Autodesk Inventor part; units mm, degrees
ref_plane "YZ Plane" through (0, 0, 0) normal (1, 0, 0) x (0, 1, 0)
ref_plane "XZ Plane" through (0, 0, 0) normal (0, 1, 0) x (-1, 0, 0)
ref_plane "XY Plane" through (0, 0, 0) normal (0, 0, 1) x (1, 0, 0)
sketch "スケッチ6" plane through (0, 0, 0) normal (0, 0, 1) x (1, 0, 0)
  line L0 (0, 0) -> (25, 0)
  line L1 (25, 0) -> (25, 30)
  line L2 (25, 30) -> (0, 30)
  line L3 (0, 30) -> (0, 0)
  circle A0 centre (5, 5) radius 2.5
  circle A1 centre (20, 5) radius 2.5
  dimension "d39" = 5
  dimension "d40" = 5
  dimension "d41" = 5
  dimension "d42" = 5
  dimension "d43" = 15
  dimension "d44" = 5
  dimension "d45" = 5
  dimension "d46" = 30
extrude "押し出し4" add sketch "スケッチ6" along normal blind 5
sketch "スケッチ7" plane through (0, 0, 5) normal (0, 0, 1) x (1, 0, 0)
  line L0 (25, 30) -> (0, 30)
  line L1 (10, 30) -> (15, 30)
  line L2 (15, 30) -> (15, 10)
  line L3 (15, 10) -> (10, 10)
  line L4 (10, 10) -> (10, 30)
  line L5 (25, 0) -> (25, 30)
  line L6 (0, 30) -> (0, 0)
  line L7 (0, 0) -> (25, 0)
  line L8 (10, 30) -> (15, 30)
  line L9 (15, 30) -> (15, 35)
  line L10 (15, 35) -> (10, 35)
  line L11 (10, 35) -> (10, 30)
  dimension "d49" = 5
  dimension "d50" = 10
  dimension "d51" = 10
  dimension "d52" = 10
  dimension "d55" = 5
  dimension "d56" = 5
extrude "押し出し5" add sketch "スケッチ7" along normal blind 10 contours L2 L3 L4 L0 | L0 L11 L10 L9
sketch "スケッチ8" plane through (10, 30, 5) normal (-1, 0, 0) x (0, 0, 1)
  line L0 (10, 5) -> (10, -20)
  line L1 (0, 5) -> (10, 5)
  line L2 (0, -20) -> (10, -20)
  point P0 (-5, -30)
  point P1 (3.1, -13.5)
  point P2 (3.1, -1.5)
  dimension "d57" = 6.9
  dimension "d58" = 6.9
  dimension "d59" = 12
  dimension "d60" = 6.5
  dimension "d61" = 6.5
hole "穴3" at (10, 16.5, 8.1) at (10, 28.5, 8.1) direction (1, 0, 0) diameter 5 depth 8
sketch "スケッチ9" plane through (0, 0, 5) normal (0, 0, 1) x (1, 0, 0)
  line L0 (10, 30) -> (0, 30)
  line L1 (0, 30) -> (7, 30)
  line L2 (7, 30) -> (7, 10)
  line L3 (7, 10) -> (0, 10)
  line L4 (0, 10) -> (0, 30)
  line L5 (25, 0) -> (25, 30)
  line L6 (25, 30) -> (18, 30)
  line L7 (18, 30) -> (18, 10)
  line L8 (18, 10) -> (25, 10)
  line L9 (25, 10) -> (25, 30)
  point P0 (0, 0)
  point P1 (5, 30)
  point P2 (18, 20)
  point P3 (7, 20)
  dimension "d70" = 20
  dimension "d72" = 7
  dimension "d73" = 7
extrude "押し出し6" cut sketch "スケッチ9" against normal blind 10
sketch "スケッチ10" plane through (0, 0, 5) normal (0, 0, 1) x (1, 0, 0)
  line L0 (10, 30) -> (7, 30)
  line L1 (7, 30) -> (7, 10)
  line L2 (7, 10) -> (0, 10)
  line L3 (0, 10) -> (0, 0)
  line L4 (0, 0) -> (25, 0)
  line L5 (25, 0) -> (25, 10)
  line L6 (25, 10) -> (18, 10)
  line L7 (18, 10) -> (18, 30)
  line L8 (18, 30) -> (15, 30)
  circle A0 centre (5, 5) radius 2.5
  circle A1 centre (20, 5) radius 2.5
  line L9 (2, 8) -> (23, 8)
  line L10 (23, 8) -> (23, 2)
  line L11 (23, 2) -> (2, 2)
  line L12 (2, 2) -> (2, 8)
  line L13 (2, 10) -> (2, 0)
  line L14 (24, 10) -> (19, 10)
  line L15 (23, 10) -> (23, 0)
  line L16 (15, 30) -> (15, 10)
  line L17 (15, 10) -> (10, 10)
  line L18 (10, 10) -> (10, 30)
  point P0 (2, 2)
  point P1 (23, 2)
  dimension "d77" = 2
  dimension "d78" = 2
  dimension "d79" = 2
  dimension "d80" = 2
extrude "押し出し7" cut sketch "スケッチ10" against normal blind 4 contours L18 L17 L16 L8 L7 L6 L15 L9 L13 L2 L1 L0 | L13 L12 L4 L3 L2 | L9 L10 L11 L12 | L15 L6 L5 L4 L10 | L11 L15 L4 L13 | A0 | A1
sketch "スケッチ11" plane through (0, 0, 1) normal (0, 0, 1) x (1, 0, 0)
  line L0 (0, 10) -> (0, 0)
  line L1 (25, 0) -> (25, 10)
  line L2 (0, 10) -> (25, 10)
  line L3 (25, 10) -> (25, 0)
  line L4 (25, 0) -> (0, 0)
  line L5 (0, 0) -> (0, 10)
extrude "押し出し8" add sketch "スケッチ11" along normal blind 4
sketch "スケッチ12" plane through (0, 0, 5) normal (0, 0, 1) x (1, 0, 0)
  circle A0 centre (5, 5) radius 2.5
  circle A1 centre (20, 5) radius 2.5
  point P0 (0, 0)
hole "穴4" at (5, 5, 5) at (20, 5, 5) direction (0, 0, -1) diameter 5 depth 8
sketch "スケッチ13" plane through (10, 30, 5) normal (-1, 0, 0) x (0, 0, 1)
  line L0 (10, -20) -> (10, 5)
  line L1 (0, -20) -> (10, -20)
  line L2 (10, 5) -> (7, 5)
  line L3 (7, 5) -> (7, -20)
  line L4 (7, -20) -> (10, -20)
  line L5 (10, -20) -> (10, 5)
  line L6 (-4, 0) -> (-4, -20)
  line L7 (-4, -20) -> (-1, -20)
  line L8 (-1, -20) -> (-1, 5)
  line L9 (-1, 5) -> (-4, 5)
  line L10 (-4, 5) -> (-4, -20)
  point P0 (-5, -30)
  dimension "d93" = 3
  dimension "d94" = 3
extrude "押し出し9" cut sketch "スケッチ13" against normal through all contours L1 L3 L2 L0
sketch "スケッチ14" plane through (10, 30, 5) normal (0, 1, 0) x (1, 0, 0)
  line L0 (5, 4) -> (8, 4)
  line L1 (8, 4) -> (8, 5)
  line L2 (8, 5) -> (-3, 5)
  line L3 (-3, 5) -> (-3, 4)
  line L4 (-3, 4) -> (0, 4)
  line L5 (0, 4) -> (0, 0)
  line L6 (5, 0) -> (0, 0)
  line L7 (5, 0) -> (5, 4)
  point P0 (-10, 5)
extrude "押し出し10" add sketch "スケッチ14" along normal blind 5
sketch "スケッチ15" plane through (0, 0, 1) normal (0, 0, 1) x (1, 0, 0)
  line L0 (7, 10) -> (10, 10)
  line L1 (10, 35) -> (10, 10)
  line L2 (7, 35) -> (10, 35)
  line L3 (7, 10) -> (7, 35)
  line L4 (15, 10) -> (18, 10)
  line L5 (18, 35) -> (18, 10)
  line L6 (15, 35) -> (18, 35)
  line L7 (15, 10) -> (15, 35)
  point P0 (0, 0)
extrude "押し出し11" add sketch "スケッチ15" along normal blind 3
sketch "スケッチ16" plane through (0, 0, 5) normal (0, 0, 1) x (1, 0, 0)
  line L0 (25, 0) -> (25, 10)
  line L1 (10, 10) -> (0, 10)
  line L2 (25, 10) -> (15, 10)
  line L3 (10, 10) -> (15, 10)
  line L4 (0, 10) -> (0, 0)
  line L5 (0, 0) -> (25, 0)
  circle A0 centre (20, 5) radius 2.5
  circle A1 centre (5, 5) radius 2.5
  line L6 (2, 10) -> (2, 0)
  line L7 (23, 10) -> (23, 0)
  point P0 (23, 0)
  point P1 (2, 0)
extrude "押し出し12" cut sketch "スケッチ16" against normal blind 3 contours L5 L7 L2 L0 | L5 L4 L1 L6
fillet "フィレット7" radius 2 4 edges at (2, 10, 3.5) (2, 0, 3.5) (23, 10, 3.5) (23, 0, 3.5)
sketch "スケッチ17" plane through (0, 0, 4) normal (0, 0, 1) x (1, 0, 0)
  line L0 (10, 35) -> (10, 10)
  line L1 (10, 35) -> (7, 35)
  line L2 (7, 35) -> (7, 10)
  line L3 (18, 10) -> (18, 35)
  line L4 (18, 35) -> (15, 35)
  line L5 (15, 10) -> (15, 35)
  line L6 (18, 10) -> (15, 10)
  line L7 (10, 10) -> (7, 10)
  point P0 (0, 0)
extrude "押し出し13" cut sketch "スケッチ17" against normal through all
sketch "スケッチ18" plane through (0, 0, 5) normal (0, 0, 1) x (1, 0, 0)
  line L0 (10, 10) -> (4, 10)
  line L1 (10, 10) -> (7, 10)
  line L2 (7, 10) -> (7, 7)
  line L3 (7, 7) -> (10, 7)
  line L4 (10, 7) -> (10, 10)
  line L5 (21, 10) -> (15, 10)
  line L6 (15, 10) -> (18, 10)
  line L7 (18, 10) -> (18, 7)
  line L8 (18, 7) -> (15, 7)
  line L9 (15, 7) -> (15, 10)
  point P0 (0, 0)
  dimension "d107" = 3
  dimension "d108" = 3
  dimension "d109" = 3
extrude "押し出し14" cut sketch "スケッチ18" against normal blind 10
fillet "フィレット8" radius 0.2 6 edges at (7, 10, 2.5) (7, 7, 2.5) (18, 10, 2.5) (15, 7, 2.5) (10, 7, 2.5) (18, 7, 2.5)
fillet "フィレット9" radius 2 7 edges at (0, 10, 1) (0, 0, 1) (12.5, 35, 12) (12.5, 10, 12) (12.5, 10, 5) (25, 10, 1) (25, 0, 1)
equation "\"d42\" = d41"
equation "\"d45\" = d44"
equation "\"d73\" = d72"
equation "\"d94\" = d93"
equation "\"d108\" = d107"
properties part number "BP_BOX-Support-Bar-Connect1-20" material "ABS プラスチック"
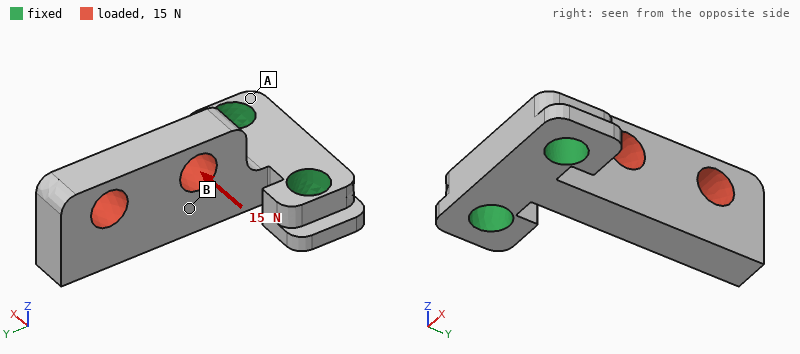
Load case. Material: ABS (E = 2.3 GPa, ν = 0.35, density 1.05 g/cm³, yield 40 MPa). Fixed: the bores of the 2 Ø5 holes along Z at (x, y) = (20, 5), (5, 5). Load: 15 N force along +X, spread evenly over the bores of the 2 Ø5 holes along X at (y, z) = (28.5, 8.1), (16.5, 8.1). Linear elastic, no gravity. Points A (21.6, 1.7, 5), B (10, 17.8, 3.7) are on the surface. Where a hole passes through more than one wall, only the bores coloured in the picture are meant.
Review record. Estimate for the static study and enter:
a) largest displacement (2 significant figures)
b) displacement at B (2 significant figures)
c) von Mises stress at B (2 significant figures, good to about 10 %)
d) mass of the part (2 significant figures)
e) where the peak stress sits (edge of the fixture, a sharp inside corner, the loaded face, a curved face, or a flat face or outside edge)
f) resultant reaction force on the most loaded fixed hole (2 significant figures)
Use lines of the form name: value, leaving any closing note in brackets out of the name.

largest displacement: 0.47 mm
displacement at B: 0.13 mm
von Mises stress at B: 3.0 MPa
mass of the part: 2.2 g
where the peak stress sits: a curved face
resultant reaction force on the most loaded fixed hole: 28 N
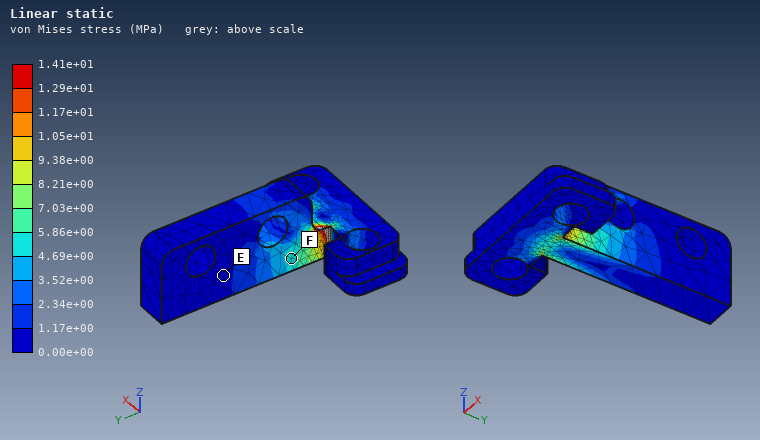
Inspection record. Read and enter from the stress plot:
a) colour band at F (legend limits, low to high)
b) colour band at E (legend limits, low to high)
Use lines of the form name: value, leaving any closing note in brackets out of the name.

colour band at F: 4.69e+00 to 5.86e+00 MPa
colour band at E: 0.00e+00 to 1.17e+00 MPa
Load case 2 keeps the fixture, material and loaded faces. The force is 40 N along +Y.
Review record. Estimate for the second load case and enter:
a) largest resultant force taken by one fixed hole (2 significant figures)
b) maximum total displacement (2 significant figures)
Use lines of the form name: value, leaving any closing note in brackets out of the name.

largest resultant force taken by one fixed hole: 20 N
maximum total displacement: 0.45 mm
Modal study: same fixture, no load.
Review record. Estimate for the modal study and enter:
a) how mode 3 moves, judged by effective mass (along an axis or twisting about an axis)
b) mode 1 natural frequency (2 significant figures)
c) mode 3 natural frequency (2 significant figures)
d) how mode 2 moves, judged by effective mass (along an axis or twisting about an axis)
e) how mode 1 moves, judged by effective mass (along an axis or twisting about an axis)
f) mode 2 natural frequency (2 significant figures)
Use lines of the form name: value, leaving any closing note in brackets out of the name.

how mode 3 moves, judged by effective mass: twisting about Y
mode 1 natural frequency: 920 Hz
mode 3 natural frequency: 3300 Hz
how mode 2 moves, judged by effective mass: along X
how mode 1 moves, judged by effective mass: along Z
mode 2 natural frequency: 990 Hz
